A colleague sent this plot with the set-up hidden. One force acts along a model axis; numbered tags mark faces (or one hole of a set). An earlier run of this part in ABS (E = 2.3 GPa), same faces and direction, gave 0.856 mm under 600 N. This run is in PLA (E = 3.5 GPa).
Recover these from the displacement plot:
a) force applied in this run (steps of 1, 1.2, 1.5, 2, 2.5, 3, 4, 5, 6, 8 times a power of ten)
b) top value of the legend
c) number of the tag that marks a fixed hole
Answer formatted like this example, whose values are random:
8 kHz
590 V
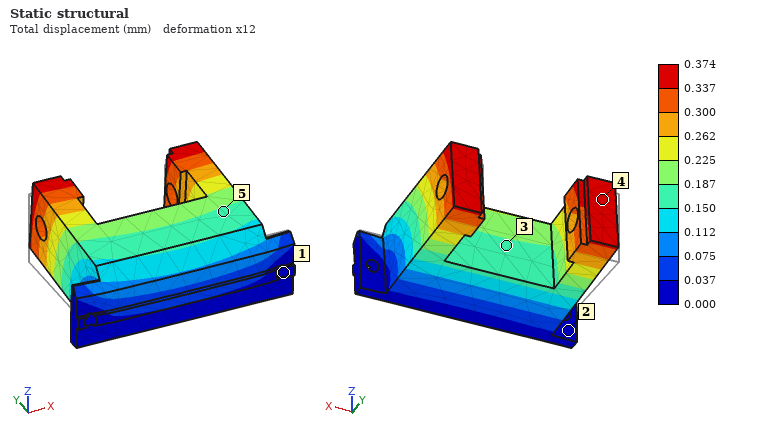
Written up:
400 N
0.374 mm
1
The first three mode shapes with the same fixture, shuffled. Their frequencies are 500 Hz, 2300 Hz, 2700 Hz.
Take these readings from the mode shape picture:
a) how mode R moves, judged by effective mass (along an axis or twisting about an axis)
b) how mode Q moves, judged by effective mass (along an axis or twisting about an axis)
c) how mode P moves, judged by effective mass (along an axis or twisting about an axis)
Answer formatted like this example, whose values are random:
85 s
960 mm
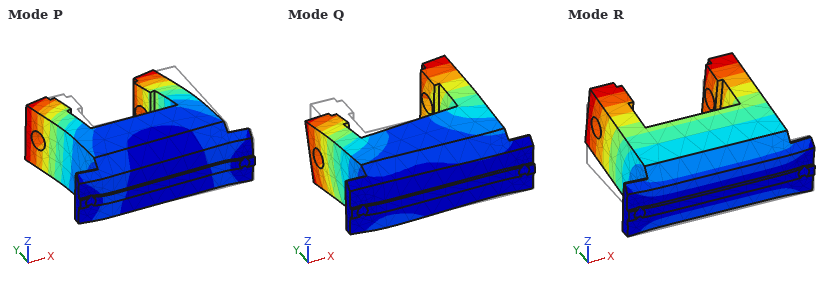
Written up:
along Z
twisting about Y
along X
